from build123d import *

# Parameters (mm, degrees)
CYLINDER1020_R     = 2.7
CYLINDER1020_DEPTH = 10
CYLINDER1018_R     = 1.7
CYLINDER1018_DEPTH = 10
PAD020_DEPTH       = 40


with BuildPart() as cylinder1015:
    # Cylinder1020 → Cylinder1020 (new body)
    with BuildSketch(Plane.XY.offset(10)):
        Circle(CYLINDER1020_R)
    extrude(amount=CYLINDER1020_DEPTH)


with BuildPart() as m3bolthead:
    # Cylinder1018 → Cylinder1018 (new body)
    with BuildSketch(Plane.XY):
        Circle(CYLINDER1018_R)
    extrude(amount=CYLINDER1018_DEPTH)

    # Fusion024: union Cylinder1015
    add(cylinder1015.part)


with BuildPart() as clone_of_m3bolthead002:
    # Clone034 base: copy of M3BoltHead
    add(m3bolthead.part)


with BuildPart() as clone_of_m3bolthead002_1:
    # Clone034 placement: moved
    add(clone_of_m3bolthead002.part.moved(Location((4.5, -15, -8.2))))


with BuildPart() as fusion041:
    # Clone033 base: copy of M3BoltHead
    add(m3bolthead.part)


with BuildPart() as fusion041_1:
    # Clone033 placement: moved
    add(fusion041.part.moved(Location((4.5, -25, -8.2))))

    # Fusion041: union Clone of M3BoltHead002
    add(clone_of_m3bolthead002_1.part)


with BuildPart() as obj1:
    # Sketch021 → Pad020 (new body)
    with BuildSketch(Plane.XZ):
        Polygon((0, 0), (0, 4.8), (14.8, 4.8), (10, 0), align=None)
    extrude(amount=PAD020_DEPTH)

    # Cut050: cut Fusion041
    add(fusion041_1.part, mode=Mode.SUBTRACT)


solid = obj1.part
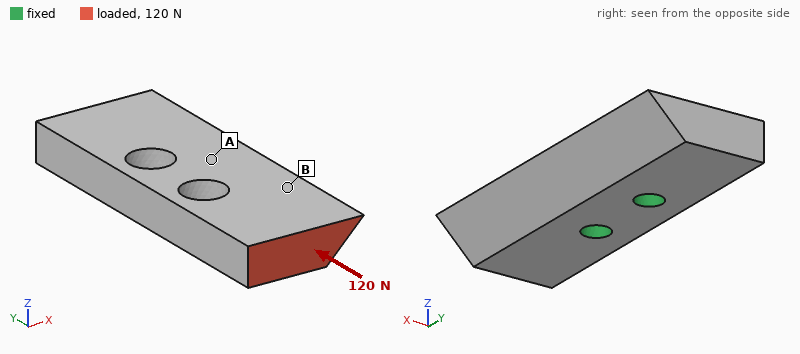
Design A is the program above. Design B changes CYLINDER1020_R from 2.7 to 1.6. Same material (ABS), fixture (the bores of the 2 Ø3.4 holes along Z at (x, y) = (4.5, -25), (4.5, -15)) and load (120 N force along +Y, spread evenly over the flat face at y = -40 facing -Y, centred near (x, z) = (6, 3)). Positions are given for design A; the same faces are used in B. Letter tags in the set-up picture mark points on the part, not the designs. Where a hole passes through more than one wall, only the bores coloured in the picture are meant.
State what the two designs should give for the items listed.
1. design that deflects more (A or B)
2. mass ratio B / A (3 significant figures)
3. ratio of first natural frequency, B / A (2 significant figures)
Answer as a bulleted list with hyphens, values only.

- A
- 1.04
- 1.2
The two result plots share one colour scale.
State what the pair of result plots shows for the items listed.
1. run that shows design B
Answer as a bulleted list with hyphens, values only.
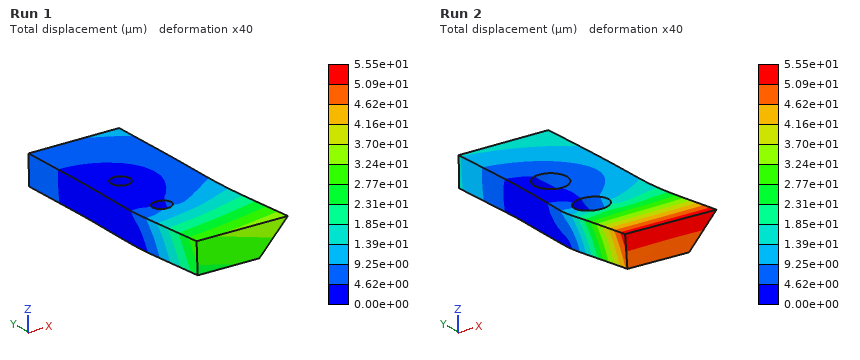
- Run 1
